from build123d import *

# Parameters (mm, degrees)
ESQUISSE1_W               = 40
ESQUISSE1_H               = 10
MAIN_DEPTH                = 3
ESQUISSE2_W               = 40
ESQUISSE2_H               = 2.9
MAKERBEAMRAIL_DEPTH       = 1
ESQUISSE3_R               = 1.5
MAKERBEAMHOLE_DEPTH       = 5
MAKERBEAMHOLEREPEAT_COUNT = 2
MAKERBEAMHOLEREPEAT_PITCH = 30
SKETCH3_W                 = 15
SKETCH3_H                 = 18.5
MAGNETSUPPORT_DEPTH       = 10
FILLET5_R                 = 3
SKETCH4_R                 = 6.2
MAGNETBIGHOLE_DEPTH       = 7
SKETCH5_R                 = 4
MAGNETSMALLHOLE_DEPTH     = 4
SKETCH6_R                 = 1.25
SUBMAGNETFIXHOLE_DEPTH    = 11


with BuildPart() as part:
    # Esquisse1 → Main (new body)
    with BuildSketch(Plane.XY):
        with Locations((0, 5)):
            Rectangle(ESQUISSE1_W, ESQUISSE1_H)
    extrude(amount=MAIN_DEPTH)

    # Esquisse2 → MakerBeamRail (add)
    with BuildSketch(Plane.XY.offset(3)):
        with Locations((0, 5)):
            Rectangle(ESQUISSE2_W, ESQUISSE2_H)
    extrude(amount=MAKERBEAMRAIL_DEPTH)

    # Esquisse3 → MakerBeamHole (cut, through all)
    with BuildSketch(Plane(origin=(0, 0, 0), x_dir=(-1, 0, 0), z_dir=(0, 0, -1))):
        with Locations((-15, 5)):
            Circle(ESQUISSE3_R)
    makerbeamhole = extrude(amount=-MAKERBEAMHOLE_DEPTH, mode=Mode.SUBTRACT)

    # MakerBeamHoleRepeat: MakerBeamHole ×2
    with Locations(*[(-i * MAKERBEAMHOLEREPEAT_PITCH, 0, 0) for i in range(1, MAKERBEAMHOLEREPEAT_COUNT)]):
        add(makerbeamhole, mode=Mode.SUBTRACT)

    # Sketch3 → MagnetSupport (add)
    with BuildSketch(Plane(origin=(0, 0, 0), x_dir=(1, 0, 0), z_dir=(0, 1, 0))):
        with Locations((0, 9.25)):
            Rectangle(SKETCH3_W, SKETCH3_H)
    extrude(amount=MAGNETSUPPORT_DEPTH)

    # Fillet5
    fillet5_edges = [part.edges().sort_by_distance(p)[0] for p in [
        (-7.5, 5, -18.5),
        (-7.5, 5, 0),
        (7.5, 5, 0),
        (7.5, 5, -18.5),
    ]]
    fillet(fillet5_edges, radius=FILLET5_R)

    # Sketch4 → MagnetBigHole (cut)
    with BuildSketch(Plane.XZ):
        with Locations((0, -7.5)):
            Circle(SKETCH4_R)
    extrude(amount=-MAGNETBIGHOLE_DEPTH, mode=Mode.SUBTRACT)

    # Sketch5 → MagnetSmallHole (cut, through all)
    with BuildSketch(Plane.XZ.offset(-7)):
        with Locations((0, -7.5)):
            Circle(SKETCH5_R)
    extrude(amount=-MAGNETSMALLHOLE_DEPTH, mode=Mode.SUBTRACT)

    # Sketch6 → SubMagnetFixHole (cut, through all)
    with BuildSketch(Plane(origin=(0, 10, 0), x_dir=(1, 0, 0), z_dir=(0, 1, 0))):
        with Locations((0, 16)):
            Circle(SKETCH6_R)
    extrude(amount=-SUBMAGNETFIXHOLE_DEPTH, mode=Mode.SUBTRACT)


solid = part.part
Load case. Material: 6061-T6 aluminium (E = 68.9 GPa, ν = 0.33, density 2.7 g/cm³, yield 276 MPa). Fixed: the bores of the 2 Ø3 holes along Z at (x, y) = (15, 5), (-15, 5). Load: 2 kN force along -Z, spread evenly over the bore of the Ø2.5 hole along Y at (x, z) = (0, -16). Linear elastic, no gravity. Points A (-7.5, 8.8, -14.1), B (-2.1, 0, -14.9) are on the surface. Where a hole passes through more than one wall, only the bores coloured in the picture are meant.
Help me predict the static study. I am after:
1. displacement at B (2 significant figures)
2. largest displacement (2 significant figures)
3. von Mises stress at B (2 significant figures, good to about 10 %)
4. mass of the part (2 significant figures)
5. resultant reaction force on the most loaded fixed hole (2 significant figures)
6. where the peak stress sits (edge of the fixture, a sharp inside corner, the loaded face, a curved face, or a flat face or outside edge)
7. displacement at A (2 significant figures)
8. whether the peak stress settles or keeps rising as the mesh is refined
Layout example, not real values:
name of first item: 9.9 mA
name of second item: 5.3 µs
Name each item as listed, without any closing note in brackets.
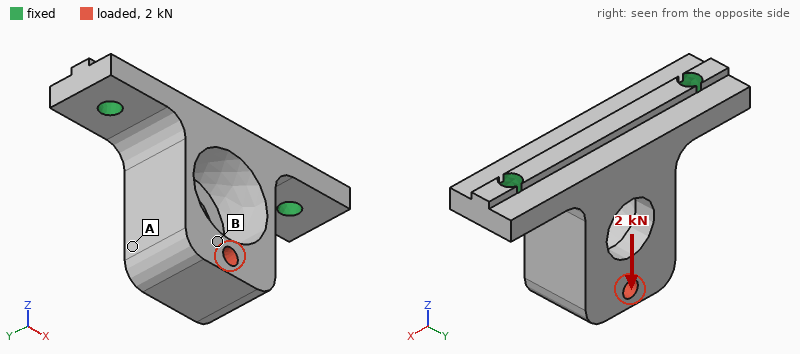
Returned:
displacement at B: 49 µm
largest displacement: 53 µm
von Mises stress at B: 60 MPa
mass of the part: 8.1 g
resultant reaction force on the most loaded fixed hole: 1.1 kN
where the peak stress sits: edge of the fixture
displacement at A: 30 µm
whether the peak stress settles or keeps rising as the mesh is refined: keeps rising
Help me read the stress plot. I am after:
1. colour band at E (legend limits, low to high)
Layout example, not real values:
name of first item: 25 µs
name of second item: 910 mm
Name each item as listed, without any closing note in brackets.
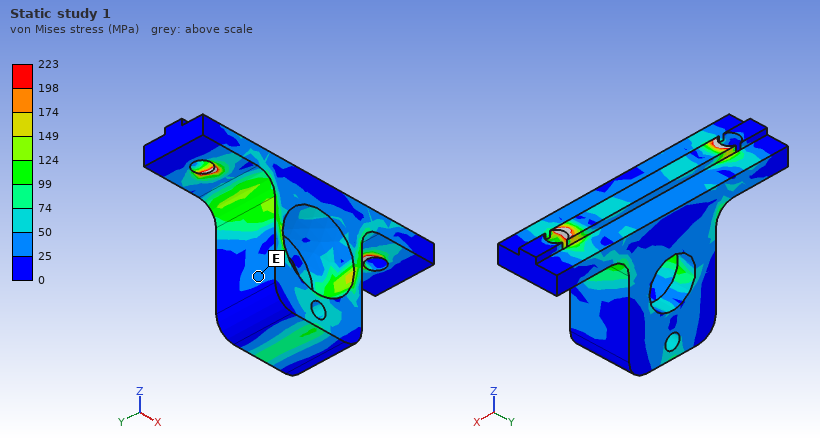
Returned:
colour band at E: 25 to 50 MPa
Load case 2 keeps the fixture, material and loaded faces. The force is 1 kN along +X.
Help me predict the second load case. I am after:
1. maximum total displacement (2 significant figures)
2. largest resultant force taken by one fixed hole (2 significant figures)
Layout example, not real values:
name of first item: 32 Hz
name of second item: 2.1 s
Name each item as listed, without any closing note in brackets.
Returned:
maximum total displacement: 0.10 mm
largest resultant force taken by one fixed hole: 920 N
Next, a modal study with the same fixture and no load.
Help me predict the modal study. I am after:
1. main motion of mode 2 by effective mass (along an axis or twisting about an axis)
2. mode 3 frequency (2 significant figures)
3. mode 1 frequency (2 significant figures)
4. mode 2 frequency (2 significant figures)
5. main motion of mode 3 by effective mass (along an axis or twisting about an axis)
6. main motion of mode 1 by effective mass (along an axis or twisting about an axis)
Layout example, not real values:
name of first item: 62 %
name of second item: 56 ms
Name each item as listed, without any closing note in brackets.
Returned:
main motion of mode 2 by effective mass: along X
mode 3 frequency: 16 kHz
mode 1 frequency: 4800 Hz
mode 2 frequency: 11 kHz
main motion of mode 3 by effective mass: along Z
main motion of mode 1 by effective mass: along Y
